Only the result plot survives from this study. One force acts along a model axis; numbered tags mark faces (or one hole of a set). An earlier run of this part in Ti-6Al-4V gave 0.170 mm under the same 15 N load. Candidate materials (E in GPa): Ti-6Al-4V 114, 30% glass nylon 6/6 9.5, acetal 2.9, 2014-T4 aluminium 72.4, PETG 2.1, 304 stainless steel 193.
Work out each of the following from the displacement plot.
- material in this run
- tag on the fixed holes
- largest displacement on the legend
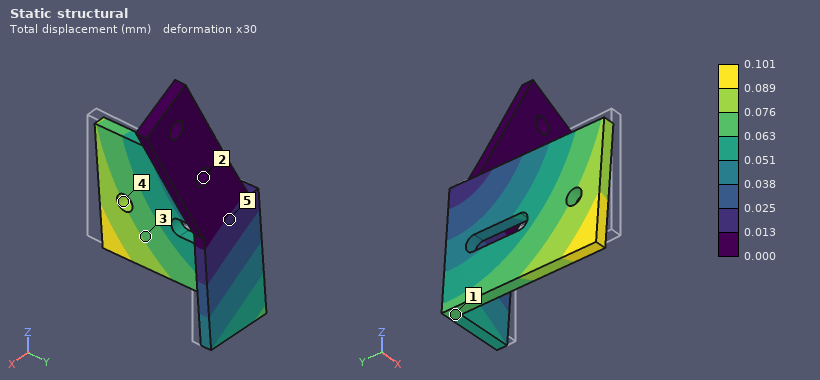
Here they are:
304 stainless steel
2
0.101 mm
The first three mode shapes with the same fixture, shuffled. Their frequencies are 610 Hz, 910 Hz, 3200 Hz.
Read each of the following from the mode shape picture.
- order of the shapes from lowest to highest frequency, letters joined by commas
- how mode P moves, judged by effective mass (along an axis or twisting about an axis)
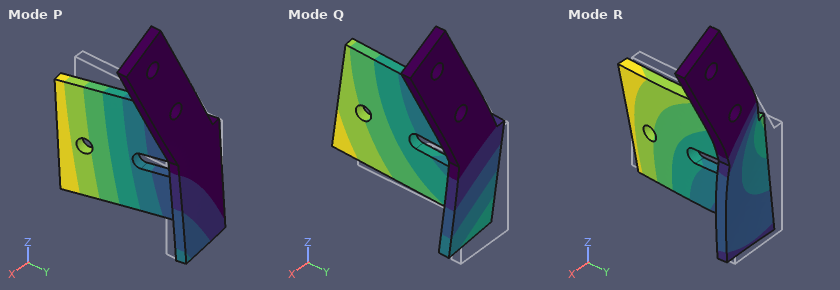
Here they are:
Q, P, R
along X
